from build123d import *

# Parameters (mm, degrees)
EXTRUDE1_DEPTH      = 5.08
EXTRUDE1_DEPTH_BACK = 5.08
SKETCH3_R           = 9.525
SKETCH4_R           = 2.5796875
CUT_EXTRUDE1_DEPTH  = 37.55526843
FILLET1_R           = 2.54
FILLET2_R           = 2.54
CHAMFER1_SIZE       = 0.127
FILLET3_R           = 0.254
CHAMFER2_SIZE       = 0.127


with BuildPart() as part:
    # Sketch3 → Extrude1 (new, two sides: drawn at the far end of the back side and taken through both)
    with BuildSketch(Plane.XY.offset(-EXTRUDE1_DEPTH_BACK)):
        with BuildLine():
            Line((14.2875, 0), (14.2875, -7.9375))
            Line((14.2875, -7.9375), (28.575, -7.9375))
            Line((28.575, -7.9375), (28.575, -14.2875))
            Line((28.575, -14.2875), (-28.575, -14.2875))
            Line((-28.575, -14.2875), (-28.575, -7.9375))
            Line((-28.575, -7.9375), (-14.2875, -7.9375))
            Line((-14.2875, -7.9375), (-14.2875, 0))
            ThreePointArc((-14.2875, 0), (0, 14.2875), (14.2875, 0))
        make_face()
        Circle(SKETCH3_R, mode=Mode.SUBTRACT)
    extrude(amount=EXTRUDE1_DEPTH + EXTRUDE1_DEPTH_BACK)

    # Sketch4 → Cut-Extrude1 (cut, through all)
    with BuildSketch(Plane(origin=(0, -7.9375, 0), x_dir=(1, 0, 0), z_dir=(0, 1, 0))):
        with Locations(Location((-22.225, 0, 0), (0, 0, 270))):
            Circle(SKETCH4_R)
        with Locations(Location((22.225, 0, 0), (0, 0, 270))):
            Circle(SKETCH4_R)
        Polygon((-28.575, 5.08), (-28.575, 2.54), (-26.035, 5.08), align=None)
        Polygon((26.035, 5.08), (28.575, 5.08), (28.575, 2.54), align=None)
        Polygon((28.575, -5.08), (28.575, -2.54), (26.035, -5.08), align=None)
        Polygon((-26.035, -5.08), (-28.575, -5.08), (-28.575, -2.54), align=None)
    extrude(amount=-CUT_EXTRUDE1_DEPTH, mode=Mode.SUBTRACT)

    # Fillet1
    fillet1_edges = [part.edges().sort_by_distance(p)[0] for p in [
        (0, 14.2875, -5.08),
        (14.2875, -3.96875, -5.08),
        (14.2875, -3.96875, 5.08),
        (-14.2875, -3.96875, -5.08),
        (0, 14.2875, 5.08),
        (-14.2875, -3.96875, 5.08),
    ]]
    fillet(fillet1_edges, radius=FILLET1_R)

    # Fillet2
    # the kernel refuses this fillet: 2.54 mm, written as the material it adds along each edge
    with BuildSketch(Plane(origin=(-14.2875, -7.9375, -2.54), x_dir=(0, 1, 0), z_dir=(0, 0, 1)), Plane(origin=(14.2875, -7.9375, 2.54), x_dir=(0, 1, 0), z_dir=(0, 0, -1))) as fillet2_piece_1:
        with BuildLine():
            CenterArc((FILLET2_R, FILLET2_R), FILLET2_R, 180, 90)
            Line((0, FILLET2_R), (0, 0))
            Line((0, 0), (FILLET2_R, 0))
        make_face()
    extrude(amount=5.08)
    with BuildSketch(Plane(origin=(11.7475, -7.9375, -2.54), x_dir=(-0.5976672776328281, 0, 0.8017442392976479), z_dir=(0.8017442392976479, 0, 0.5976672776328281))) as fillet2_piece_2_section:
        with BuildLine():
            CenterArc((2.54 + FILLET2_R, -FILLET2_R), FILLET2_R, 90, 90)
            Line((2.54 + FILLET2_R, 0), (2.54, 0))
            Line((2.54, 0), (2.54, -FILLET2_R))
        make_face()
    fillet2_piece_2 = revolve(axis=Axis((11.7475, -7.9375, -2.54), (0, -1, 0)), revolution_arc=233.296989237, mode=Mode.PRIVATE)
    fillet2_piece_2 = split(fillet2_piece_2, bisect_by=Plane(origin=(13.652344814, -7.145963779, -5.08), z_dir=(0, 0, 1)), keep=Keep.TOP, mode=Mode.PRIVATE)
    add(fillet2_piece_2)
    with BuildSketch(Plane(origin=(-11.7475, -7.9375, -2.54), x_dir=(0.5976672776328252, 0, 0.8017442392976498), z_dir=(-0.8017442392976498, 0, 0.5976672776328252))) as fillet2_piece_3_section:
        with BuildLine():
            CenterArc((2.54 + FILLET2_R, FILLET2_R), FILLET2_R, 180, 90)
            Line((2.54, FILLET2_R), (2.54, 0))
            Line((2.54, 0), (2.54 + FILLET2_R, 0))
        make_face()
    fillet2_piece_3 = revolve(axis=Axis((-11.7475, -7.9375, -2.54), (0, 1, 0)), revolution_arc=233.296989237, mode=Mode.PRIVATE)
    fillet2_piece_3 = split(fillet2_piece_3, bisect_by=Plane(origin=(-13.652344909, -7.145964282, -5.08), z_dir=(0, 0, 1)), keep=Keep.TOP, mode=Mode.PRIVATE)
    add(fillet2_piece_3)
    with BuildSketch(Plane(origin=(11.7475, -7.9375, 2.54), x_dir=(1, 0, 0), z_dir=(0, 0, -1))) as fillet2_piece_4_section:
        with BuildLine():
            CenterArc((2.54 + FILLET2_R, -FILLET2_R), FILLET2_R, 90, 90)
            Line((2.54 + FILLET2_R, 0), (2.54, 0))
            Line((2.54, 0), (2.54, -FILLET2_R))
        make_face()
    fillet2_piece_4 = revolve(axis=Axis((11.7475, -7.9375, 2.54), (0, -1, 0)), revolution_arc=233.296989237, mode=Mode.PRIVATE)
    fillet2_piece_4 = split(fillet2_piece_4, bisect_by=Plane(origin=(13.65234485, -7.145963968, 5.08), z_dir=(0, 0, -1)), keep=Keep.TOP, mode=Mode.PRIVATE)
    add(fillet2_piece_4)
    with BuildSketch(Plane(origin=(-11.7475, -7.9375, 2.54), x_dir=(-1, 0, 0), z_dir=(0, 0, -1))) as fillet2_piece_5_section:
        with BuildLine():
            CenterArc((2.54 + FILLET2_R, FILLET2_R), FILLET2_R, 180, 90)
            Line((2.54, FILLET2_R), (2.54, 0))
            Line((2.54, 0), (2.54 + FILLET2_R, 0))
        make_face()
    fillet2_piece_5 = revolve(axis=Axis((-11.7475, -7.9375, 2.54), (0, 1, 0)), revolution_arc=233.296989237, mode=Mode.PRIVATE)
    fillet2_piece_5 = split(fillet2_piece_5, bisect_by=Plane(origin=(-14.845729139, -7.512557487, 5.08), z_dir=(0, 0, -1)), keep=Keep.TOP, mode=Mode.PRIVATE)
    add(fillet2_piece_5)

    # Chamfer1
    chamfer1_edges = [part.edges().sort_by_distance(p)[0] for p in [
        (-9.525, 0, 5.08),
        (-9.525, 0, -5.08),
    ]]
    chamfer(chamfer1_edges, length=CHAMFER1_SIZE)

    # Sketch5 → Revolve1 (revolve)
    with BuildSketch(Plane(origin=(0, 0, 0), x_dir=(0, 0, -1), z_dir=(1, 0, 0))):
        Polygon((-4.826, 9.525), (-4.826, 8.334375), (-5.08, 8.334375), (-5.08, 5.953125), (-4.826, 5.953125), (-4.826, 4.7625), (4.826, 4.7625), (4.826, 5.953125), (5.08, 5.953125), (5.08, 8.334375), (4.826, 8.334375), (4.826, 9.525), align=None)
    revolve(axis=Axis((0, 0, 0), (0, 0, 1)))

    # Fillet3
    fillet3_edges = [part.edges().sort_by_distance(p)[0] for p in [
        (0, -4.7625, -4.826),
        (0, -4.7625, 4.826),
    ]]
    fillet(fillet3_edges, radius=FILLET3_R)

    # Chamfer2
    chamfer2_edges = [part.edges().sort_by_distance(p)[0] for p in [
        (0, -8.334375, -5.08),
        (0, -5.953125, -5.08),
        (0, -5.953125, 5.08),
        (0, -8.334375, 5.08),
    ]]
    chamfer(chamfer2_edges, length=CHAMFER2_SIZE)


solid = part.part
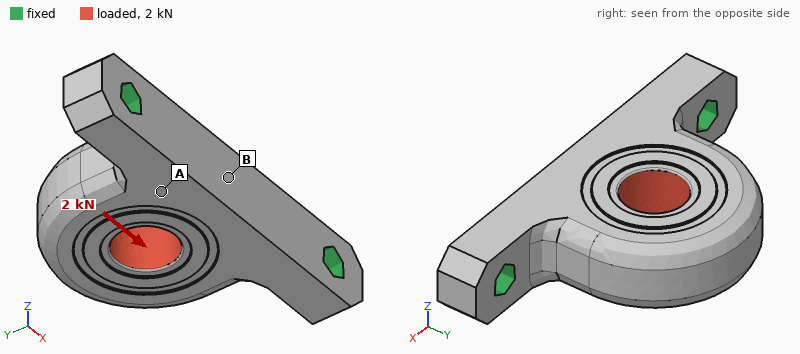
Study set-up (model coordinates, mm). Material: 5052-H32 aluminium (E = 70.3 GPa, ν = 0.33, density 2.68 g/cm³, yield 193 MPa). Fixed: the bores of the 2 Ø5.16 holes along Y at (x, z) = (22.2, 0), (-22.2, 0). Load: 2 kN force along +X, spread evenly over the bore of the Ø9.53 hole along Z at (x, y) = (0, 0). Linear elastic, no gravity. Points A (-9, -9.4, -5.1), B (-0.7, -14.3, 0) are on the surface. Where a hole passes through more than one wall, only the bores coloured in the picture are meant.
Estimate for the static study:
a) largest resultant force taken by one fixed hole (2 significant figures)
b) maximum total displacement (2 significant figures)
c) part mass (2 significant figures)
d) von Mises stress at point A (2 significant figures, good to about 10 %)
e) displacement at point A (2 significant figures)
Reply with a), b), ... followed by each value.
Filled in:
a) 1.2 kN
b) 12 µm
c) 21 g
d) 9.5 MPa
e) 3.0 µm
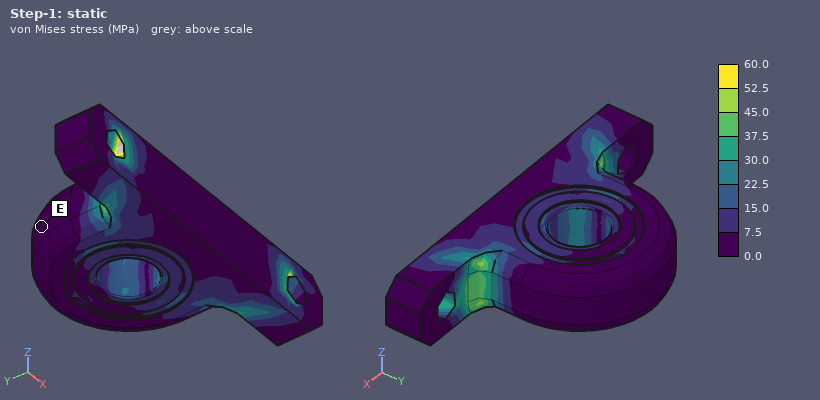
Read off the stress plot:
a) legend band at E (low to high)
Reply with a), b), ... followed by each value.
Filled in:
a) 0.0 to 7.5 MPa
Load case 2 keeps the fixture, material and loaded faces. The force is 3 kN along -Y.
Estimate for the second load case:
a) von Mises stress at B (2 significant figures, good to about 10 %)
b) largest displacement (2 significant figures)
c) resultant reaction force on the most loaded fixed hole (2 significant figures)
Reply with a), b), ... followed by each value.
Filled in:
a) 26 MPa
b) 20 µm
c) 1.7 kN
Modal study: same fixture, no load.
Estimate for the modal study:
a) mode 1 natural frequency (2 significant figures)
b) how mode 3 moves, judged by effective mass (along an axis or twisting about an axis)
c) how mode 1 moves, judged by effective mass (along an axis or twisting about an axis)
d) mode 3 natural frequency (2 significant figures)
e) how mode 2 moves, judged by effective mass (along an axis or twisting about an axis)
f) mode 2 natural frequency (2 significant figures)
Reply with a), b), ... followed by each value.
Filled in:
a) 5500 Hz
b) along X
c) along Z
d) 18 kHz
e) along Y
f) 16 kHz
